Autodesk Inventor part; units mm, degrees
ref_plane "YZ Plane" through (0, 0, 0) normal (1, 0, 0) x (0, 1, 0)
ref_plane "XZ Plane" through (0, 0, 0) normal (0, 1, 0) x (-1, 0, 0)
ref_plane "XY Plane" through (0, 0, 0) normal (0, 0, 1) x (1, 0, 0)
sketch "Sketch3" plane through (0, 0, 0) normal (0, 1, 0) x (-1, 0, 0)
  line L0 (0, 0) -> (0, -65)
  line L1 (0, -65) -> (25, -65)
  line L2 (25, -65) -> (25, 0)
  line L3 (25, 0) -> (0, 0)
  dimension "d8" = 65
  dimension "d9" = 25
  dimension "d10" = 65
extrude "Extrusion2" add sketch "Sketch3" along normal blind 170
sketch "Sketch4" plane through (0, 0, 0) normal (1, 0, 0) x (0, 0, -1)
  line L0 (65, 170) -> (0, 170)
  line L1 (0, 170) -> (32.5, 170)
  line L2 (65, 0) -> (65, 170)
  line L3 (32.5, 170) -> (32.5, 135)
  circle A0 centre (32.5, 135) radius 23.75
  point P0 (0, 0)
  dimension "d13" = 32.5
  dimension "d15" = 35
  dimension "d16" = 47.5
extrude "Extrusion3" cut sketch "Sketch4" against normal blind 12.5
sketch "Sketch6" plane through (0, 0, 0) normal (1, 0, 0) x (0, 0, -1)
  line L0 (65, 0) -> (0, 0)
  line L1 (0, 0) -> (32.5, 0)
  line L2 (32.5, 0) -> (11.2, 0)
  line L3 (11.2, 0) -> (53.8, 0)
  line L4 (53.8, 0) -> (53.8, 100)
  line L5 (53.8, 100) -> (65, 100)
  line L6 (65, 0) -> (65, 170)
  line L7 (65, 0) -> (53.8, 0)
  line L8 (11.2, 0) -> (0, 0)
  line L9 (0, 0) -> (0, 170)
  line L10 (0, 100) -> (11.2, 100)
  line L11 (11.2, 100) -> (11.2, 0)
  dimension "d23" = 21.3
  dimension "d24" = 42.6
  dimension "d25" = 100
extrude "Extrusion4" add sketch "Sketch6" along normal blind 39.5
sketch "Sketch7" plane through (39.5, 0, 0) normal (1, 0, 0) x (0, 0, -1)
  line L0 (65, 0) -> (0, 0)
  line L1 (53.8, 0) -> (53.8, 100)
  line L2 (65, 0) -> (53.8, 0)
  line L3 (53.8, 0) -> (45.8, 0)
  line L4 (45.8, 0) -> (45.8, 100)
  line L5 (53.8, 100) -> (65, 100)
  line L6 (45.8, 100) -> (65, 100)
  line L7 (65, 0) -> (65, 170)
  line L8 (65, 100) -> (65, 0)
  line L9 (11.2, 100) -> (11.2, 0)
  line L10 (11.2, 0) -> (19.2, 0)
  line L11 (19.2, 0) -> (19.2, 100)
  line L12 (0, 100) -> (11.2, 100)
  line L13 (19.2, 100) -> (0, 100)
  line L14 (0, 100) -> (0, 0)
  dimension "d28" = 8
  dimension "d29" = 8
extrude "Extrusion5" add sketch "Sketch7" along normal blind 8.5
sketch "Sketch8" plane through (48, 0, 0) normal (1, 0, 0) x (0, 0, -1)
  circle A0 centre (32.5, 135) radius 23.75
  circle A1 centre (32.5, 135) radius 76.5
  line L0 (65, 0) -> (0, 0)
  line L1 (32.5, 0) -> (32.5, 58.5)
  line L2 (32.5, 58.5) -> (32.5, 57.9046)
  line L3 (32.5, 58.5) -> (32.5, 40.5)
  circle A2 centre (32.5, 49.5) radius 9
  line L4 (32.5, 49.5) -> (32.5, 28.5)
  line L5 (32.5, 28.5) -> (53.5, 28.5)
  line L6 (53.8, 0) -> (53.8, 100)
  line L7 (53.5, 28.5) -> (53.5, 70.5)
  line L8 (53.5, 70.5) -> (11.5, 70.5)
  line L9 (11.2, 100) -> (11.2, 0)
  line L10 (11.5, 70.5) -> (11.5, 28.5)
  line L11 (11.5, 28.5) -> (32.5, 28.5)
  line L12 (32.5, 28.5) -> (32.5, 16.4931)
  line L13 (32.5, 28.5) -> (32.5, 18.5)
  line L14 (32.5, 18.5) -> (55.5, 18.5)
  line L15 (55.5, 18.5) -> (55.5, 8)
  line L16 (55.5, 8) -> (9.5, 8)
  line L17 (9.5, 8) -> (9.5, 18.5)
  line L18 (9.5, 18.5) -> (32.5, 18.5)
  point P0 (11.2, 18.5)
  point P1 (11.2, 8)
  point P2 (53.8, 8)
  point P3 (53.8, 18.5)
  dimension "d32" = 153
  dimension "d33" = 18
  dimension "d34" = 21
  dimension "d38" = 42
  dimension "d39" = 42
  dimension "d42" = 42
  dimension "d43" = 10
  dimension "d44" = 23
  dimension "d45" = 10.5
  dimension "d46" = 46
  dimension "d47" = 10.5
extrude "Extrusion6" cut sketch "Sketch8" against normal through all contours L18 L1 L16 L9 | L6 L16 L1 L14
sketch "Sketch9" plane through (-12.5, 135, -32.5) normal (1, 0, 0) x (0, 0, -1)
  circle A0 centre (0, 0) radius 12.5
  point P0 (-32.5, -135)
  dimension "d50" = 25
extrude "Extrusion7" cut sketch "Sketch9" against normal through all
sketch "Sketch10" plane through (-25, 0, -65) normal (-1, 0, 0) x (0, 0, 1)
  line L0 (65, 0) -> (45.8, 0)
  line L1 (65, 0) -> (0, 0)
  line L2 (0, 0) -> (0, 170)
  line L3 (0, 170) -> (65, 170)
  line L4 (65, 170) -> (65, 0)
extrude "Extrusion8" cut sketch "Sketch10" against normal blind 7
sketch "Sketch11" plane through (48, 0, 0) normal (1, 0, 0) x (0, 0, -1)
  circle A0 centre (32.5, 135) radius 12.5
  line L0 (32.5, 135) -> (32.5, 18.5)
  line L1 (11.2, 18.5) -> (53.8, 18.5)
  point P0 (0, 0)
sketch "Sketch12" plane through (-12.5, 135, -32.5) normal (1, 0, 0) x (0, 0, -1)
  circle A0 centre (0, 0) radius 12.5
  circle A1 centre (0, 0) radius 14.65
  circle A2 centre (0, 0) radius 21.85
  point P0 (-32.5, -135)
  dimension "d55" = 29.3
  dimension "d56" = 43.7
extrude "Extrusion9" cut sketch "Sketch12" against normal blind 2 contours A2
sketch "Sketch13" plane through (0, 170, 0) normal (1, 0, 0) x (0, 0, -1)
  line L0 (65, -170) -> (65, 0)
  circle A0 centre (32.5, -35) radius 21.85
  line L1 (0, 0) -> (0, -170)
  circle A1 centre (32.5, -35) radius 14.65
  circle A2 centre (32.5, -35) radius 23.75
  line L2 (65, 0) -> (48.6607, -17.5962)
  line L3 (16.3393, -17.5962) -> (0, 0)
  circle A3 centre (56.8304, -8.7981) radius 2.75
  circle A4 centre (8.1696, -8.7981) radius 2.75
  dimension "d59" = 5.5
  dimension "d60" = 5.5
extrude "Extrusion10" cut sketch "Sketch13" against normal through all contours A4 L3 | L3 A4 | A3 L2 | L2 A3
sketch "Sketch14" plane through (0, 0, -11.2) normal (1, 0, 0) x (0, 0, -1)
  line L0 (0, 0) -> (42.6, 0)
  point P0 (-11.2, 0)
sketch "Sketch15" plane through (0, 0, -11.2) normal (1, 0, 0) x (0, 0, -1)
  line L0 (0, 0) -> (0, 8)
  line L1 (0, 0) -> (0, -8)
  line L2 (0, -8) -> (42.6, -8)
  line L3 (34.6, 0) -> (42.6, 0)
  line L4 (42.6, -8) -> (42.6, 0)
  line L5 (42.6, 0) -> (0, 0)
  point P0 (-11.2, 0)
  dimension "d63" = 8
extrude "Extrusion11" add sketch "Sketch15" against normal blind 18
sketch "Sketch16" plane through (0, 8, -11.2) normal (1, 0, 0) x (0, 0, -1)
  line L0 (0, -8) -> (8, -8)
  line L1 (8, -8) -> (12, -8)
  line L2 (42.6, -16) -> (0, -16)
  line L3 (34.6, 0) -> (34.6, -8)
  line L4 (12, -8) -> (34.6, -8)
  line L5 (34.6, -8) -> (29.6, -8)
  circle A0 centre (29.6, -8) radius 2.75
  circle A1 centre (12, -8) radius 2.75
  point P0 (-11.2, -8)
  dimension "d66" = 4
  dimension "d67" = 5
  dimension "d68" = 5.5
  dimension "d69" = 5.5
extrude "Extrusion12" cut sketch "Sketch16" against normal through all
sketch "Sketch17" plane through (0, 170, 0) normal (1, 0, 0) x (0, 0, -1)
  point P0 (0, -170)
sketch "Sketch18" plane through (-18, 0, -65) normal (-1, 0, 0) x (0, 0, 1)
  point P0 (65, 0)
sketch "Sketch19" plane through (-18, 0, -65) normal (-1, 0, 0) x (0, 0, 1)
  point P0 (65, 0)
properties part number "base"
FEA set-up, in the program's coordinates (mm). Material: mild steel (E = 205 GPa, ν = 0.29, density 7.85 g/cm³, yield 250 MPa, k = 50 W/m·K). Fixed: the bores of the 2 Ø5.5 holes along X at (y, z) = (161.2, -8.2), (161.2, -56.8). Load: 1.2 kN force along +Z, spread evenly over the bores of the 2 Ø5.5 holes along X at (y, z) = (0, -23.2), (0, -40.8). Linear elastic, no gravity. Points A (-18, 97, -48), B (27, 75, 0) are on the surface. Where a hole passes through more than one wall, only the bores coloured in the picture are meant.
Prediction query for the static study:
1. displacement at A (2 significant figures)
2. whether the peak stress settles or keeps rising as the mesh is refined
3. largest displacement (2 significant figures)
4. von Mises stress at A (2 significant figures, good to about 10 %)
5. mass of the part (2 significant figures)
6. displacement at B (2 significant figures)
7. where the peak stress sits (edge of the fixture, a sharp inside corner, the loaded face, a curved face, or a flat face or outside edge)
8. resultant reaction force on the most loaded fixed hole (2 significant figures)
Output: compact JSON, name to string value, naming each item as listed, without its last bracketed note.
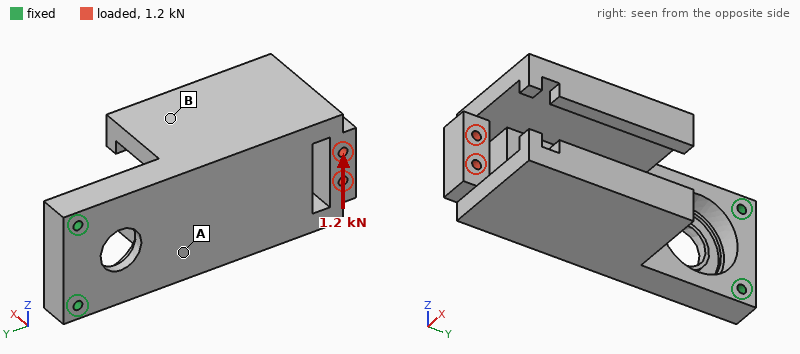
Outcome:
{"displacement at A": "10 µm", "whether the peak stress settles or keeps rising as the mesh is refined": "keeps rising", "largest displacement": "35 µm", "von Mises stress at A": "5.4 MPa", "mass of the part": "2.3 kg", "displacement at B": "17 µm", "where the peak stress sits": "edge of the fixture", "resultant reaction force on the most loaded fixed hole": "3.7 kN"}
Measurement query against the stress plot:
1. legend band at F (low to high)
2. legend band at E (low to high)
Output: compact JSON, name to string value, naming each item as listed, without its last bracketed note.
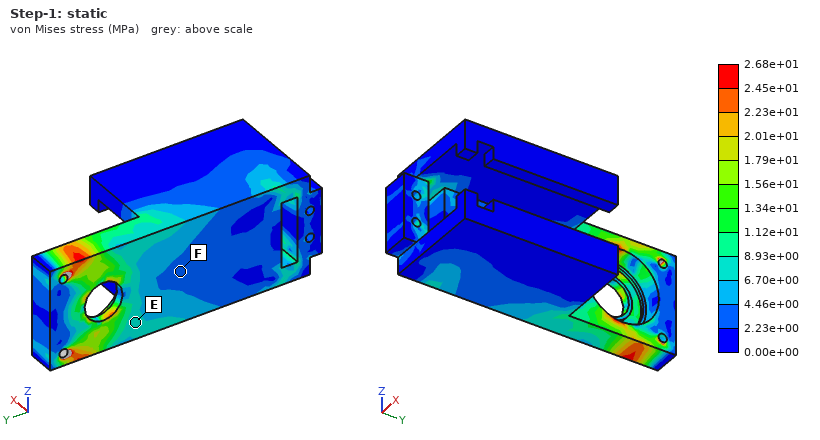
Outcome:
{"legend band at F": "2.23e+00 to 4.46e+00 MPa", "legend band at E": "6.70e+00 to 8.93e+00 MPa"}
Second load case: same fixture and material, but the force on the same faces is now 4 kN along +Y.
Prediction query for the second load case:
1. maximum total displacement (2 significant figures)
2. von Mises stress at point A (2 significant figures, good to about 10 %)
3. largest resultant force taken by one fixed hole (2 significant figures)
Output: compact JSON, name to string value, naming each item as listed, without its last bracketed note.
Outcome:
{"maximum total displacement": "17 µm", "von Mises stress at point A": "3.7 MPa", "largest resultant force taken by one fixed hole": "2.0 kN"}
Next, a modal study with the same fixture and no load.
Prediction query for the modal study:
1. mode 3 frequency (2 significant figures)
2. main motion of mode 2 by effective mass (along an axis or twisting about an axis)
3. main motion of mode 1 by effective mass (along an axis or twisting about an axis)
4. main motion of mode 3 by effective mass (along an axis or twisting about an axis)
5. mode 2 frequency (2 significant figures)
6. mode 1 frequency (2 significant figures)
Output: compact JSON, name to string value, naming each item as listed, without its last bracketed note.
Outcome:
{"mode 3 frequency": "1400 Hz", "main motion of mode 2 by effective mass": "along Z", "main motion of mode 1 by effective mass": "along X", "main motion of mode 3 by effective mass": "along Z", "mode 2 frequency": "730 Hz", "mode 1 frequency": "280 Hz"}
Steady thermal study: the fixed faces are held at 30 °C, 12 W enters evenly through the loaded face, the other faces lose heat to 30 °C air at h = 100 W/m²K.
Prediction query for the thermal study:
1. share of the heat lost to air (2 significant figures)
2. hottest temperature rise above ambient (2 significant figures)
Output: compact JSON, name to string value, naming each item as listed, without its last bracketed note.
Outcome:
{"share of the heat lost to air": "98 %", "hottest temperature rise above ambient": "15 K"}
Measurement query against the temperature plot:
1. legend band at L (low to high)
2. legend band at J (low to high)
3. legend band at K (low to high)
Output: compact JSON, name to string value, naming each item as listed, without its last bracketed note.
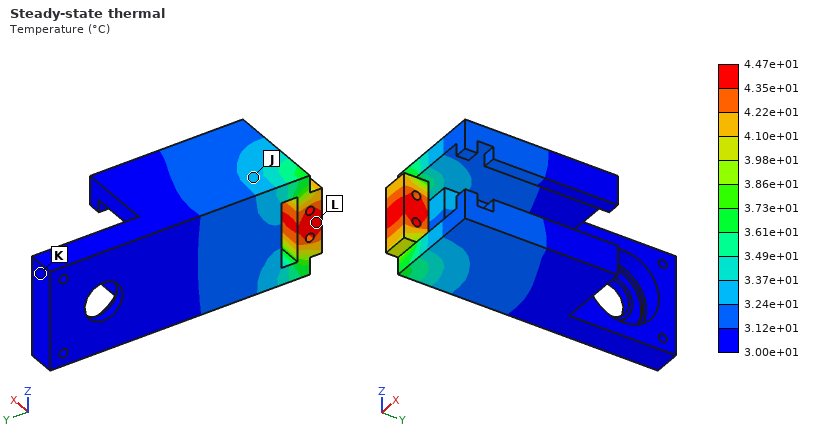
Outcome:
{"legend band at L": "4.35e+01 to 4.47e+01 °C", "legend band at J": "3.24e+01 to 3.37e+01 °C", "legend band at K": "3.00e+01 to 3.12e+01 °C"}
